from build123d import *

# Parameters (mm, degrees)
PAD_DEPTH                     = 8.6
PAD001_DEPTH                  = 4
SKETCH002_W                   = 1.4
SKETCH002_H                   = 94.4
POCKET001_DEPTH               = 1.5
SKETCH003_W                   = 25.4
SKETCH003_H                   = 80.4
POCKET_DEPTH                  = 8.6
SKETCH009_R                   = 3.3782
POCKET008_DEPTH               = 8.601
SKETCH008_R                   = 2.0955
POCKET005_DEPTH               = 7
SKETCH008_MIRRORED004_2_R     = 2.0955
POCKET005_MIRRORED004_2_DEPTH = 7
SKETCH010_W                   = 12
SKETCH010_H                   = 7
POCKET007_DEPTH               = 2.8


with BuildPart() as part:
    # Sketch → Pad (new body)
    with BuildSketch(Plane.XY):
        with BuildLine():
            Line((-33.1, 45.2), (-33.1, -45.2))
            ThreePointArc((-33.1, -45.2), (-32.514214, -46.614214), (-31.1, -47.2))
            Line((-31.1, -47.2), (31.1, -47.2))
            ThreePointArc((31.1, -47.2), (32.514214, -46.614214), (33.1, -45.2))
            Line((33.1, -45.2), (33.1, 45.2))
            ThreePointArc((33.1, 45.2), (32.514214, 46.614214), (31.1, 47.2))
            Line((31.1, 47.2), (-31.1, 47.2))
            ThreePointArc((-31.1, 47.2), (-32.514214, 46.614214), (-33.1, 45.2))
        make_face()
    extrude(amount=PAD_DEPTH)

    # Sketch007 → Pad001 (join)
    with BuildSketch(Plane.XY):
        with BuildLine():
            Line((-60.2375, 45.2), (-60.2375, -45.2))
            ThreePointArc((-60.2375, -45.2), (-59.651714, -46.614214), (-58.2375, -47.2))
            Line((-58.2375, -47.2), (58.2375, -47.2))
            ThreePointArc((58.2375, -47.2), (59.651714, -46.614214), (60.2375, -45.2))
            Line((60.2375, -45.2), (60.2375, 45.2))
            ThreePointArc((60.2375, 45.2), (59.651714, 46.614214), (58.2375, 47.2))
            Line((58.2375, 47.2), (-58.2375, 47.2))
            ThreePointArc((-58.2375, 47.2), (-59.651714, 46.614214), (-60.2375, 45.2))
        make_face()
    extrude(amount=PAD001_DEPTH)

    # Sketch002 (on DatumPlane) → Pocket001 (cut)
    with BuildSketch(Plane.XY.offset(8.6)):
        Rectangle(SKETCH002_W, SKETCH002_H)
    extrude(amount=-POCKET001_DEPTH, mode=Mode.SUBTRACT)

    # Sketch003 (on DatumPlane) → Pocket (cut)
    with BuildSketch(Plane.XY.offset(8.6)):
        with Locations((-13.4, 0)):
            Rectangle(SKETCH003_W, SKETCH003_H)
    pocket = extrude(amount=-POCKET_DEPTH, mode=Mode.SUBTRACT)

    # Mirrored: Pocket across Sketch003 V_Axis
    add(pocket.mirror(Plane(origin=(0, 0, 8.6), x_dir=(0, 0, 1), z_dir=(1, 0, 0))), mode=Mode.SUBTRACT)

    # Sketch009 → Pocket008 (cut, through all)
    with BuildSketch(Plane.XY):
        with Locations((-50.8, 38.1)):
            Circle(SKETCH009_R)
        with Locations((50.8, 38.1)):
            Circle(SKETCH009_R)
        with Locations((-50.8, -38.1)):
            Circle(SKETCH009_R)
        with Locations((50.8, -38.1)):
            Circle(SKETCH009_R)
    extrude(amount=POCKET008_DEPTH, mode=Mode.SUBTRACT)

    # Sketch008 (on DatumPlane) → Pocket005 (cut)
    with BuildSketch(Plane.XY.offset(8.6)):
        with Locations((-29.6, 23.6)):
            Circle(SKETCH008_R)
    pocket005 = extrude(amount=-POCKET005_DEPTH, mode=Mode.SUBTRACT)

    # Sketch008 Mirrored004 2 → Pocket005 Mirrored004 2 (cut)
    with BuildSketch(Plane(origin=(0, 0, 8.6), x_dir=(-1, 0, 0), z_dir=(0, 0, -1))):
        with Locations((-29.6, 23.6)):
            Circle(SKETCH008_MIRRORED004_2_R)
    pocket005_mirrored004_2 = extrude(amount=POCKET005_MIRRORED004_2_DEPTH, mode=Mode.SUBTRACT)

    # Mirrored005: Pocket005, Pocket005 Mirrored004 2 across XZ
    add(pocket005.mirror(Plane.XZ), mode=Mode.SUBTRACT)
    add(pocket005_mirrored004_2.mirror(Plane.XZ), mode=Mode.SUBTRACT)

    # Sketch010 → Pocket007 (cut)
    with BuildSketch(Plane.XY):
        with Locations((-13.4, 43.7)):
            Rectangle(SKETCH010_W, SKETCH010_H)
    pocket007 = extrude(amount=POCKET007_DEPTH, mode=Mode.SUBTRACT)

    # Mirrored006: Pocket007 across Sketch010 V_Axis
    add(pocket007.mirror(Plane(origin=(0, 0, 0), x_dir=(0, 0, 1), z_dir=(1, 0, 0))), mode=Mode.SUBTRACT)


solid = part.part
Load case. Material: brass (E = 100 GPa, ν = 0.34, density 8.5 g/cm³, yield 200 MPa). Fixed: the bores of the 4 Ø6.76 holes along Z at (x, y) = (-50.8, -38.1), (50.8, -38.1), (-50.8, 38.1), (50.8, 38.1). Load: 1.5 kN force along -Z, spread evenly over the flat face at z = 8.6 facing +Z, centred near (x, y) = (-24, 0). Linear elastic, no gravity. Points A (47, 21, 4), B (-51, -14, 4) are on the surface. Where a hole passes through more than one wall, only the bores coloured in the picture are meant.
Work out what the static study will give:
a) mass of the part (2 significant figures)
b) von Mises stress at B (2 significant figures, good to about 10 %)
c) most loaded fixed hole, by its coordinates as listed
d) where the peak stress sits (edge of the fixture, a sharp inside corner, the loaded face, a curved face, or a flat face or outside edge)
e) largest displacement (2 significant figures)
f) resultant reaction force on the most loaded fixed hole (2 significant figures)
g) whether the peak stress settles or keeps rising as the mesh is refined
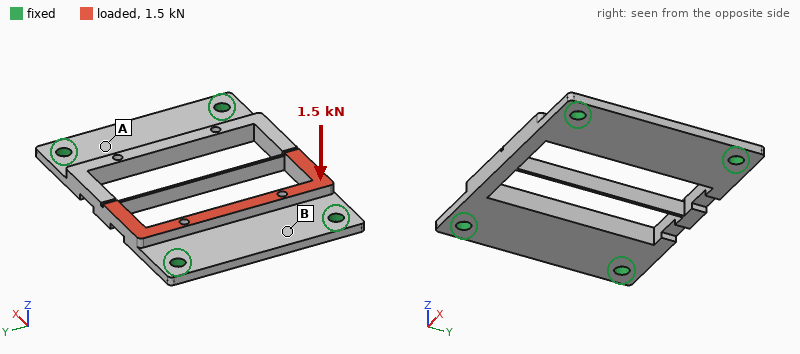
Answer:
320 g
19 MPa
(-50.8, 38.1)
edge of the fixture
0.11 mm
920 N
keeps rising
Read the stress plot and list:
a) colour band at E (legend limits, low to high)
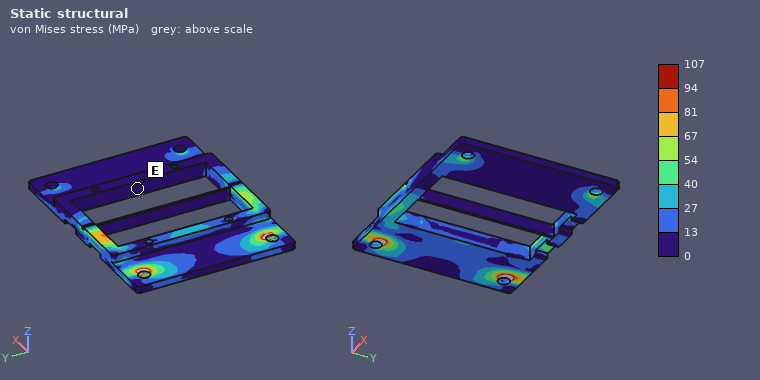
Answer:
0 to 13 MPa
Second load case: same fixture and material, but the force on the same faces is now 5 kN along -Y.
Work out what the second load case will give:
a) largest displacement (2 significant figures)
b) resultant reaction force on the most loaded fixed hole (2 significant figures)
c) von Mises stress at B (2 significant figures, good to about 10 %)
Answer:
82 µm
2.6 kN
18 MPa
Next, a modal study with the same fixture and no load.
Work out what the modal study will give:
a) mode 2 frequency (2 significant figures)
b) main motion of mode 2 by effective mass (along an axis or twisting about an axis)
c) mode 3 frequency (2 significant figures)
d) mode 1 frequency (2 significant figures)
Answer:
1800 Hz
along Z
2100 Hz
760 Hz
